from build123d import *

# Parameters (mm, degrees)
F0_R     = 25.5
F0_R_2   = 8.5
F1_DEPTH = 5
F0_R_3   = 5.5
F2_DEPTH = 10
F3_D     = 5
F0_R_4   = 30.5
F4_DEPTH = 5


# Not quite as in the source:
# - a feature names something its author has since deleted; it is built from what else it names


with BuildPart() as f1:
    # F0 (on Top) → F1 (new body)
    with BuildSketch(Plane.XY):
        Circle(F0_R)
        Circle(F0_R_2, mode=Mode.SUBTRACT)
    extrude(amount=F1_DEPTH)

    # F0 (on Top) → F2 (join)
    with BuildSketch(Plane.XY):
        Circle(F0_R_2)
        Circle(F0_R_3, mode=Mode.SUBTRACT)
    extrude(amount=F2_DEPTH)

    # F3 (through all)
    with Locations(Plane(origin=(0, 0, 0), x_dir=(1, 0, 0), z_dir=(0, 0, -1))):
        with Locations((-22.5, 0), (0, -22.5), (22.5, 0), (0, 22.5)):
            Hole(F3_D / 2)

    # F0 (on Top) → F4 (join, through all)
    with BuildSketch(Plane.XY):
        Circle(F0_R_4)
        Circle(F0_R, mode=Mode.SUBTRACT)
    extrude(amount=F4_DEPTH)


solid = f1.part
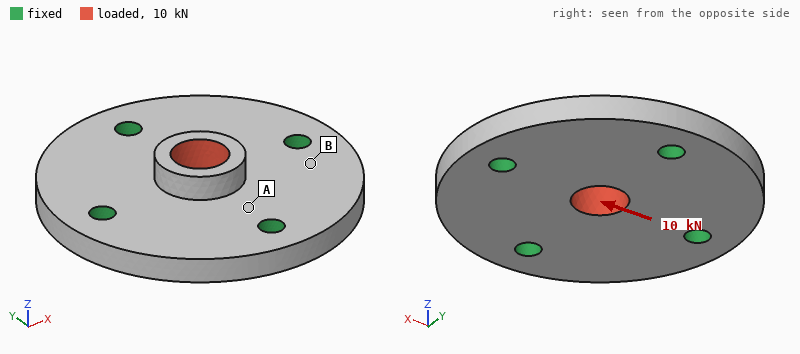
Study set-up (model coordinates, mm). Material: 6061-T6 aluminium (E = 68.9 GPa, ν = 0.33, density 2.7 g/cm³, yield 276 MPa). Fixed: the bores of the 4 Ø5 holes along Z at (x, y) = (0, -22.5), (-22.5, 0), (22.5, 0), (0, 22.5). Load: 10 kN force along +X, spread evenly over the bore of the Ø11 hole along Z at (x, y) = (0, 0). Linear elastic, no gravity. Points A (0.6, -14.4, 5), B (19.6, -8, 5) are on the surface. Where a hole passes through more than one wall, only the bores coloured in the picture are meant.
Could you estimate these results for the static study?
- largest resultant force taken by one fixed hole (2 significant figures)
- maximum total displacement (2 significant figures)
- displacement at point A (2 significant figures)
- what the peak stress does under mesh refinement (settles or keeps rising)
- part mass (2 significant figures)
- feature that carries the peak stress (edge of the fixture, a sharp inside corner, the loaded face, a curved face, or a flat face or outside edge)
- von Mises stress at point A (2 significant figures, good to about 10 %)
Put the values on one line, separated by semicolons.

3.3 kN; 33 µm; 6.0 µm; keeps rising; 39 g; edge of the fixture; 28 MPa
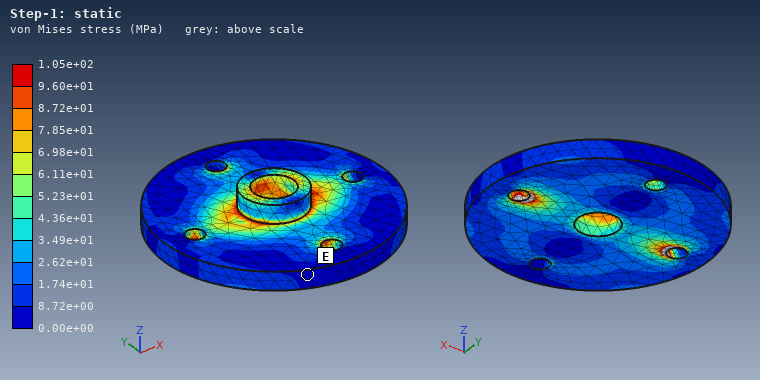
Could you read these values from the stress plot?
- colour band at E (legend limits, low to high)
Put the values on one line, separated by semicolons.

0.00e+00 to 8.72e+00 MPa
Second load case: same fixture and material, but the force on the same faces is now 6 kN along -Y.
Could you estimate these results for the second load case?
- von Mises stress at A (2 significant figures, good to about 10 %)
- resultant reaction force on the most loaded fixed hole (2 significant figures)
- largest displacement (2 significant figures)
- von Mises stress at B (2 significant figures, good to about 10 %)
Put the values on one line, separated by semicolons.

41 MPa; 2.0 kN; 20 µm; 8.4 MPa
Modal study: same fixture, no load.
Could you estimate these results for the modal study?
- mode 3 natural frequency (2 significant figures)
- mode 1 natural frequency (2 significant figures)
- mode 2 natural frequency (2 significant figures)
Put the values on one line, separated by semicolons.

17 kHz; 16 kHz; 17 kHz
